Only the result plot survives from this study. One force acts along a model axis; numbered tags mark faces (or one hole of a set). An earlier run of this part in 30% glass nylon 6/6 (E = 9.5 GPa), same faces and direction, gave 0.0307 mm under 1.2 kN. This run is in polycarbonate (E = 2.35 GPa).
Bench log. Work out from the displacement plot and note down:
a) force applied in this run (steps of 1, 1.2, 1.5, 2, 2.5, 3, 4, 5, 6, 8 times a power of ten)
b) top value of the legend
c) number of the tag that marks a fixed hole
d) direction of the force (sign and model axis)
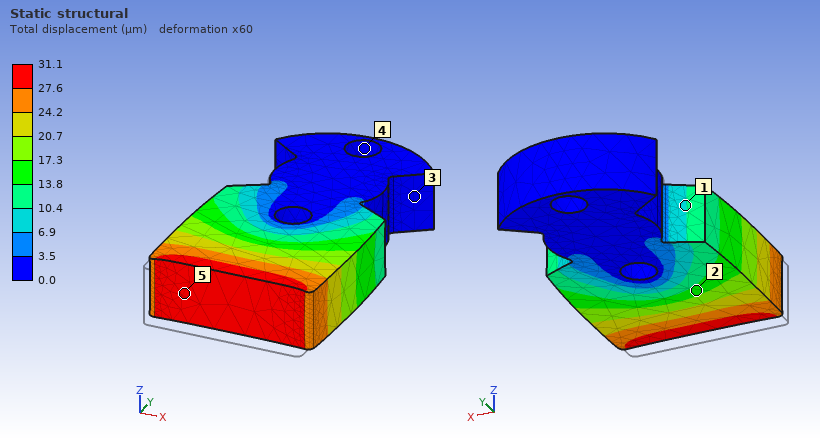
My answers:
300 N
31.1 µm
4
+Y
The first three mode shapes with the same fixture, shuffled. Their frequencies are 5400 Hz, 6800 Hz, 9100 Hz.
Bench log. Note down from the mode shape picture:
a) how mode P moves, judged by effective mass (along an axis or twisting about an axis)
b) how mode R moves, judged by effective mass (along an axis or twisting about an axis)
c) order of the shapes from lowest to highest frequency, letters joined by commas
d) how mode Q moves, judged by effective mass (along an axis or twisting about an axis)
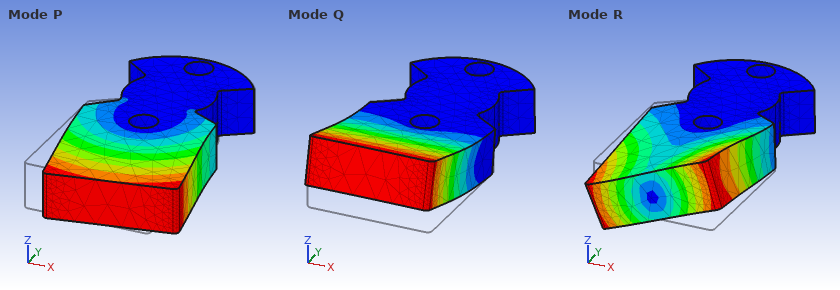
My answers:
along X
twisting about Y
Q, P, R
along Z
